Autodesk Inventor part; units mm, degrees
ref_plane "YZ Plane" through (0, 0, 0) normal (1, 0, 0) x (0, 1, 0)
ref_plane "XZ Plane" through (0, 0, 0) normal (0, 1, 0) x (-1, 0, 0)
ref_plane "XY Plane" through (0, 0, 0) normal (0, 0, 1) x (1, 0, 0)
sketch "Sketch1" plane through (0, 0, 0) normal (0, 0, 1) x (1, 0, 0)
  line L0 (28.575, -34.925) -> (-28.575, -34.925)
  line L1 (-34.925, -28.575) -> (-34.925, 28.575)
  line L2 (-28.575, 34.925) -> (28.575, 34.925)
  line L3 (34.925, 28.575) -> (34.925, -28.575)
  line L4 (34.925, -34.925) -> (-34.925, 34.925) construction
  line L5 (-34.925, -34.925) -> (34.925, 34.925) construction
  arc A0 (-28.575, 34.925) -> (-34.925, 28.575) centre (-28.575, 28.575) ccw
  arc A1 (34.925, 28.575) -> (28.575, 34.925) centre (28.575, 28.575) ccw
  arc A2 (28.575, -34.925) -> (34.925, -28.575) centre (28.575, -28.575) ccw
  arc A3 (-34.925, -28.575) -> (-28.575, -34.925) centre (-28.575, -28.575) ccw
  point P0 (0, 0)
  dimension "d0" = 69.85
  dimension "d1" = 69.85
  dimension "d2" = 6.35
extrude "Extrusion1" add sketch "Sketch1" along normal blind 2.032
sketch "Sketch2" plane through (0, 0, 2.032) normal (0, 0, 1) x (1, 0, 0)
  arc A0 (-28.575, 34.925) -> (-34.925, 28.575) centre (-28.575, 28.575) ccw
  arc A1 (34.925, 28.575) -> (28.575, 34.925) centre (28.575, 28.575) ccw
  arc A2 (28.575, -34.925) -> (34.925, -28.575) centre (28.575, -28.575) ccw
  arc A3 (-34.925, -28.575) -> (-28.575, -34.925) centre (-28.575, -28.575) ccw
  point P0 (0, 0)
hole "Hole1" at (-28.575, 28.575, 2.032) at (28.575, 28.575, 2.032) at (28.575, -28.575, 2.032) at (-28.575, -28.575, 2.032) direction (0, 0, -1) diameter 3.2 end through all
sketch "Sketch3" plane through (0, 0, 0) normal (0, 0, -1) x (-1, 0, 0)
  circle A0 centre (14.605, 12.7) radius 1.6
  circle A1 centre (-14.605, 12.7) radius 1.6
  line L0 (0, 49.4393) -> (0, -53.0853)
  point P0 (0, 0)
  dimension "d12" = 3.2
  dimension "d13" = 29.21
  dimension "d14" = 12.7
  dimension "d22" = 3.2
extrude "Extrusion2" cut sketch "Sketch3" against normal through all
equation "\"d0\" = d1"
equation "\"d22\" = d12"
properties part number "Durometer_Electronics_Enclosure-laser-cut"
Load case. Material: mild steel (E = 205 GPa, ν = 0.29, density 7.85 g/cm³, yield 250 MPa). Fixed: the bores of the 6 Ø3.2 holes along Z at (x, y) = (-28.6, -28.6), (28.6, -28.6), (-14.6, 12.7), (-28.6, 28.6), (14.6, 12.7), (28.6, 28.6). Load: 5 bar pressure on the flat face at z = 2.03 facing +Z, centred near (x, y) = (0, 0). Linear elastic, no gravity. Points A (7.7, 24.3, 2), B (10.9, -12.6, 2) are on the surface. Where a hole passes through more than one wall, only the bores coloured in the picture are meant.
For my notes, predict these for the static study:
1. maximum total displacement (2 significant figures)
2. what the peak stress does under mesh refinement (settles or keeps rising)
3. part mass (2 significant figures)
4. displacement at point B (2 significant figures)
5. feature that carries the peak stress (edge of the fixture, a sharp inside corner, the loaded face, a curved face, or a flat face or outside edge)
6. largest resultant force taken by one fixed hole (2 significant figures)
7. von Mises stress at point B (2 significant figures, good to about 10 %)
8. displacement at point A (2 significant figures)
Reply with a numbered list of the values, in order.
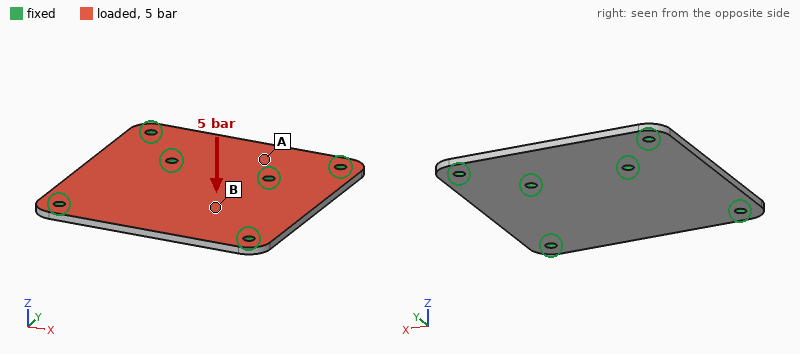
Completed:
1. 98 µm
2. keeps rising
3. 77 g
4. 70 µm
5. edge of the fixture
6. 580 N
7. 62 MPa
8. 17 µm
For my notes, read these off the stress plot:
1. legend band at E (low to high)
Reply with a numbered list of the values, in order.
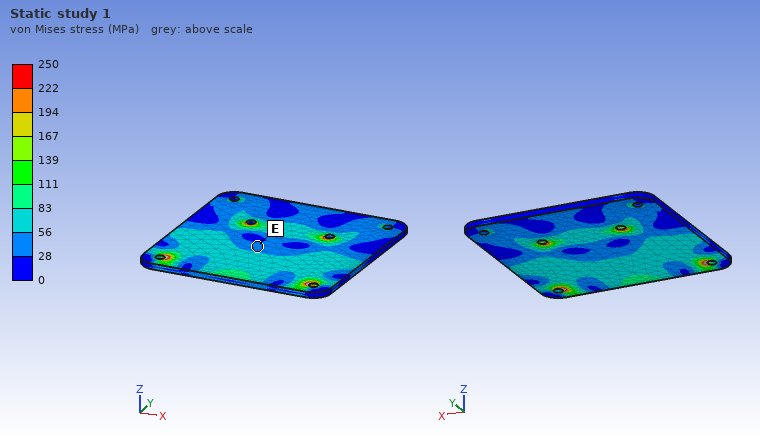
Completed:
1. 28 to 56 MPa
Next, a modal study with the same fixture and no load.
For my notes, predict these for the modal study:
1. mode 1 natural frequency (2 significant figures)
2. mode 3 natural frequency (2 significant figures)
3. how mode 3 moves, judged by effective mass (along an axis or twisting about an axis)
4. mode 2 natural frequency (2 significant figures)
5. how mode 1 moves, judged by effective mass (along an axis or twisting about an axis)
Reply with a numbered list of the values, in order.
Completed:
1. 3400 Hz
2. 5000 Hz
3. twisting about Y
4. 4700 Hz
5. along Z
